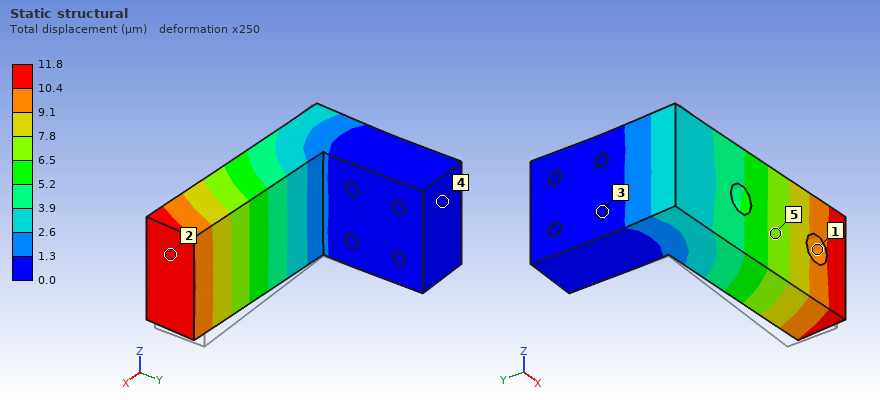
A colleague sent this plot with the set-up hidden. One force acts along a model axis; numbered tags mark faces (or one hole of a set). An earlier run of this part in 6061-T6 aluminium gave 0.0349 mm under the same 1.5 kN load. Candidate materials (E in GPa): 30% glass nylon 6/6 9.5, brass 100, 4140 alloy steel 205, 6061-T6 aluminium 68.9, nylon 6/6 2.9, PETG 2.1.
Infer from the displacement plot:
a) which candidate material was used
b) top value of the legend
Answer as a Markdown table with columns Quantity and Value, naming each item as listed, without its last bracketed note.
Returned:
| Quantity | Value |
|---|---|
| which candidate material was used | 4140 alloy steel |
| top value of the legend | 11.8 µm |
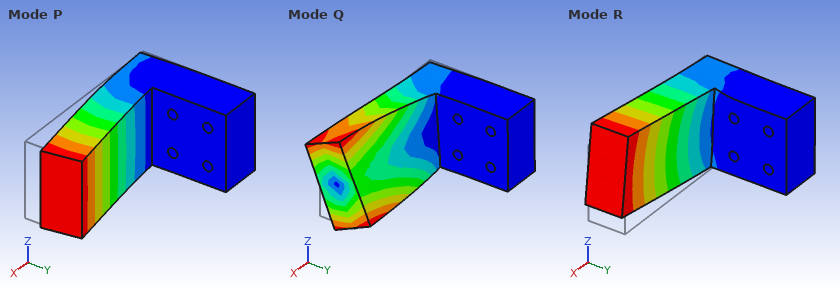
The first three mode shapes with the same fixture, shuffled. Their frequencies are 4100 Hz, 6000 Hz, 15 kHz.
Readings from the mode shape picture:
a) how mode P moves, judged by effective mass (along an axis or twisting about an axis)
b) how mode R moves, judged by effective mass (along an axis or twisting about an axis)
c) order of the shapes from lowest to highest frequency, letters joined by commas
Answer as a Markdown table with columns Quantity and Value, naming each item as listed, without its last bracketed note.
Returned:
| Quantity | Value |
|---|---|
| how mode P moves, judged by effective mass | along Y |
| how mode R moves, judged by effective mass | along Z |
| order of the shapes from lowest to highest frequency, letters joined by commas | P, R, Q |
